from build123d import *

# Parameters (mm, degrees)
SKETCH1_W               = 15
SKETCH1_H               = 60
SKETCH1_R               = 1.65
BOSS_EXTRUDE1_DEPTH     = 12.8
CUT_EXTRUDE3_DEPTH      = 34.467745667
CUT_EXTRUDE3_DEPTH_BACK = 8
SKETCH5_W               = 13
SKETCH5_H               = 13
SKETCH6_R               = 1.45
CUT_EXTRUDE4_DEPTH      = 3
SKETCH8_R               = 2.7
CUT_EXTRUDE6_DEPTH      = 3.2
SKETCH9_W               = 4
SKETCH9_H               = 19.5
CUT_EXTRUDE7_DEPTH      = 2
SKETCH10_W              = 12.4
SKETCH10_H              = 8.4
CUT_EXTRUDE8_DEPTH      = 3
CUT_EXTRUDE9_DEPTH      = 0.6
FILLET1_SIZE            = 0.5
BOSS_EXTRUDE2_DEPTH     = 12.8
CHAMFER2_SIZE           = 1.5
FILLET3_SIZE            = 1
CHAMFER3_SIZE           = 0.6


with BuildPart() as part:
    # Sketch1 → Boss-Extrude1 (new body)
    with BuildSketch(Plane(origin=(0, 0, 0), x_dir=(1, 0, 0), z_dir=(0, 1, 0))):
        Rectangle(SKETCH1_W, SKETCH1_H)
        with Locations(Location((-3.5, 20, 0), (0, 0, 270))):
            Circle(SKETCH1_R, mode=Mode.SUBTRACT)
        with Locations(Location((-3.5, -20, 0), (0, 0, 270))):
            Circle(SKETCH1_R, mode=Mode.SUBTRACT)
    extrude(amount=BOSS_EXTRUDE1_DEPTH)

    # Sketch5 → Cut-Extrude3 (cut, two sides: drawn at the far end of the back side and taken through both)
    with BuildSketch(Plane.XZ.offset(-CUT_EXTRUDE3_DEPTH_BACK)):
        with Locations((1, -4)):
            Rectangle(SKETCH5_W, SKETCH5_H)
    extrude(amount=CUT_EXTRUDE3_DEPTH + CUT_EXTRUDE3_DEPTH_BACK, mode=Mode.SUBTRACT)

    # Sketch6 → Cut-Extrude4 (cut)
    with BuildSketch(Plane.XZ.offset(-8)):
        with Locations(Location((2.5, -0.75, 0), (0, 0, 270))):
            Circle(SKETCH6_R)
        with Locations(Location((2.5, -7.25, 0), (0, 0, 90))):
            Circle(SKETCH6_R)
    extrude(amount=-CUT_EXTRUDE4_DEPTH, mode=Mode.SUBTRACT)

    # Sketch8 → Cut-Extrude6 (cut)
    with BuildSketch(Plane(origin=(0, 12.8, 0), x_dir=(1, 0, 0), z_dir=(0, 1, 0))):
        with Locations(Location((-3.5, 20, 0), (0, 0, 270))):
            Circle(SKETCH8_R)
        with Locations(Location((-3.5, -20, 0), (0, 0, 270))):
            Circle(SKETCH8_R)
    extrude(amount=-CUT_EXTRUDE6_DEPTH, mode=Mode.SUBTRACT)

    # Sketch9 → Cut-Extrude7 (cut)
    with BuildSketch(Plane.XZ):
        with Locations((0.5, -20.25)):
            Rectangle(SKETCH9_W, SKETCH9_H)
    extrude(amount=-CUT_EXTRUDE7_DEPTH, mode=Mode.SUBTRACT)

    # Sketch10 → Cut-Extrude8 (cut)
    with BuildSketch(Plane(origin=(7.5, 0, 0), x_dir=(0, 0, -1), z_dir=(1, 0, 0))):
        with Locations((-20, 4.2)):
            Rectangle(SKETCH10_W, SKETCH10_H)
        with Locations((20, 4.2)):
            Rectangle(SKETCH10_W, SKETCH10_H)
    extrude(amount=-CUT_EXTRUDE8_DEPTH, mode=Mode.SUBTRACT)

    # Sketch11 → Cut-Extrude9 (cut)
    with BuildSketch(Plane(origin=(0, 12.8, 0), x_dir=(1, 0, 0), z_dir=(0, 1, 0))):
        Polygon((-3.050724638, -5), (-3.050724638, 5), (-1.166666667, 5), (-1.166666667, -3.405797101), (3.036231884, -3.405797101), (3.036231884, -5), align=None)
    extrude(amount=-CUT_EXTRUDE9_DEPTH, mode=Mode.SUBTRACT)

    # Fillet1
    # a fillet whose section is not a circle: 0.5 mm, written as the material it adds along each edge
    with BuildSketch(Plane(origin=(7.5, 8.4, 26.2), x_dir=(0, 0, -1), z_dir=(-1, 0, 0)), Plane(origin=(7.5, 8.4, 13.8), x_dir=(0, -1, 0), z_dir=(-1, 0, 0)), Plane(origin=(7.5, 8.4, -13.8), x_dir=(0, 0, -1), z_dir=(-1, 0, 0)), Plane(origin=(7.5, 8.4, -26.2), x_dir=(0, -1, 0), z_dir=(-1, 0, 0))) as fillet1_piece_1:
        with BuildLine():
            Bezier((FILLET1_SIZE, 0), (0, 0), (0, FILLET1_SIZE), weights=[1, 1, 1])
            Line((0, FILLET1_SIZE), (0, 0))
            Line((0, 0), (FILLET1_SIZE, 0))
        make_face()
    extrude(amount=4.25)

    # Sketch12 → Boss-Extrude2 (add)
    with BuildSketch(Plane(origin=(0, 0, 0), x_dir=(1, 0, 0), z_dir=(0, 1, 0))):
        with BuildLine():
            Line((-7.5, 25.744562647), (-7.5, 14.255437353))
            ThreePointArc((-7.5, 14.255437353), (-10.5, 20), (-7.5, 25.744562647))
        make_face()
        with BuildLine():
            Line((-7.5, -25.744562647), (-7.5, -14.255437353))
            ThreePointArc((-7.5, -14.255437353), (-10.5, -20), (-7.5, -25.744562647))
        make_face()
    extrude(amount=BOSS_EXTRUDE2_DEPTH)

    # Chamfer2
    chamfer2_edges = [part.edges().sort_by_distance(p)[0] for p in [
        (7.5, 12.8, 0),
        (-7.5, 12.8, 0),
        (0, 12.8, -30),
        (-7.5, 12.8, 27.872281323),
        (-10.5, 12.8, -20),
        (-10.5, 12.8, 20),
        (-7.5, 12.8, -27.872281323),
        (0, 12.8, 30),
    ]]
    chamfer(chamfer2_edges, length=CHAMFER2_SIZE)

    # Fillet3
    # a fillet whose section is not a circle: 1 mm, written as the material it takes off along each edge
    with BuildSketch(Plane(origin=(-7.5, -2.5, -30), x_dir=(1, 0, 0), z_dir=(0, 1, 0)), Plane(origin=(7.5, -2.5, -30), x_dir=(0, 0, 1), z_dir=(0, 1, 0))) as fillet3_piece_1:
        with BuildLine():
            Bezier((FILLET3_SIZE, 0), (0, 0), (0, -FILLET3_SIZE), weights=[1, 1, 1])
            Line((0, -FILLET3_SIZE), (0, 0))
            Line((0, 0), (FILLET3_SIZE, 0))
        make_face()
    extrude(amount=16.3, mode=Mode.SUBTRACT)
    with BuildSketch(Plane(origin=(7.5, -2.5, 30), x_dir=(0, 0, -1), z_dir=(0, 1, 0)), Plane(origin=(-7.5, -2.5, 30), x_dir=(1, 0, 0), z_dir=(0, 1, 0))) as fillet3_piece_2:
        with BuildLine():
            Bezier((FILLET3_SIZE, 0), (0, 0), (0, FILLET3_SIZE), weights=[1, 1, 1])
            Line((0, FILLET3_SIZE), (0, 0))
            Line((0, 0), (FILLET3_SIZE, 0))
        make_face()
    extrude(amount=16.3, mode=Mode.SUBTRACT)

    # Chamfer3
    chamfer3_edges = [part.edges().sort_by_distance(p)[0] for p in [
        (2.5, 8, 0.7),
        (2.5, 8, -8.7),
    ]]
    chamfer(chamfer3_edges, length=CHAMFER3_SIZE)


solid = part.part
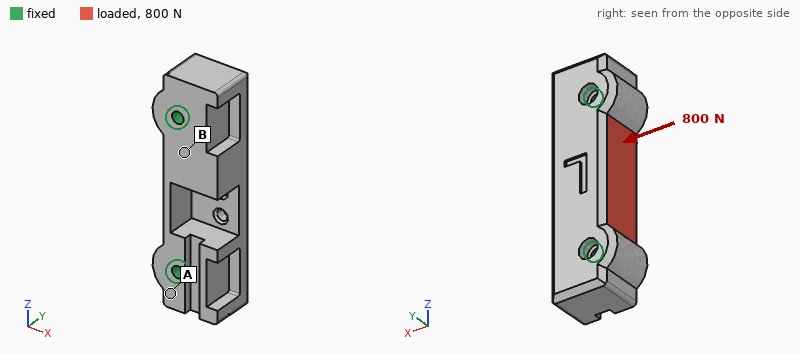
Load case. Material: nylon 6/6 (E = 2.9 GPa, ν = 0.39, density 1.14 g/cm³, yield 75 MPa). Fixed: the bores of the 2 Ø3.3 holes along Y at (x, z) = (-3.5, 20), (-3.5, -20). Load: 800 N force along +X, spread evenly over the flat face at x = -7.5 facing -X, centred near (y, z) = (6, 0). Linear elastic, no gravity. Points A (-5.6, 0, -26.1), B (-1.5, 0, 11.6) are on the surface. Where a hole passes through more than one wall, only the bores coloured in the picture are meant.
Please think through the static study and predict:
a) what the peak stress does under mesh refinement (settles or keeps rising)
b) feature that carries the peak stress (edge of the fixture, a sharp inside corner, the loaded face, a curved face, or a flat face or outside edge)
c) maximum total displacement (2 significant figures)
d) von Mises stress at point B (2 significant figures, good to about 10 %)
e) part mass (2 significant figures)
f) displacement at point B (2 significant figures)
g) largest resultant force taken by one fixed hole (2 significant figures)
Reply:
keeps rising
edge of the fixture
0.30 mm
6.5 MPa
11 g
0.079 mm
410 N
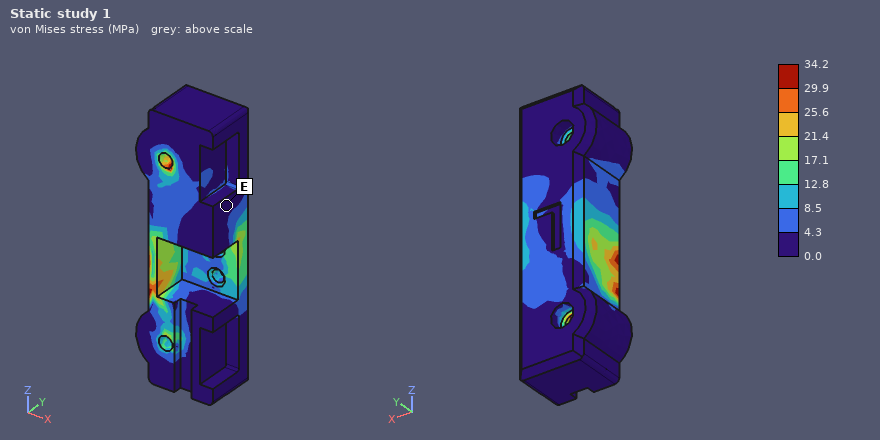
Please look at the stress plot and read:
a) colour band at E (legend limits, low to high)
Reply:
0.0 to 4.3 MPa
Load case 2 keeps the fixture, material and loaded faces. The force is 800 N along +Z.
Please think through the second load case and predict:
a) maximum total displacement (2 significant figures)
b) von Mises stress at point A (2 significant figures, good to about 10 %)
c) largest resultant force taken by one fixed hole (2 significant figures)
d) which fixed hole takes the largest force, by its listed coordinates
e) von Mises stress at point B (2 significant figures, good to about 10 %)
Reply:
43 µm
0.80 MPa
440 N
(-3.5, 20)
2.1 MPa
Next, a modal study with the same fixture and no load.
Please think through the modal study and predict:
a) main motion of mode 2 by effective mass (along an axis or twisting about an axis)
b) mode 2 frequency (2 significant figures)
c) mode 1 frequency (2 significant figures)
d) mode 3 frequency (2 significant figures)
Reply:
along Y
6800 Hz
5600 Hz
8700 Hz
